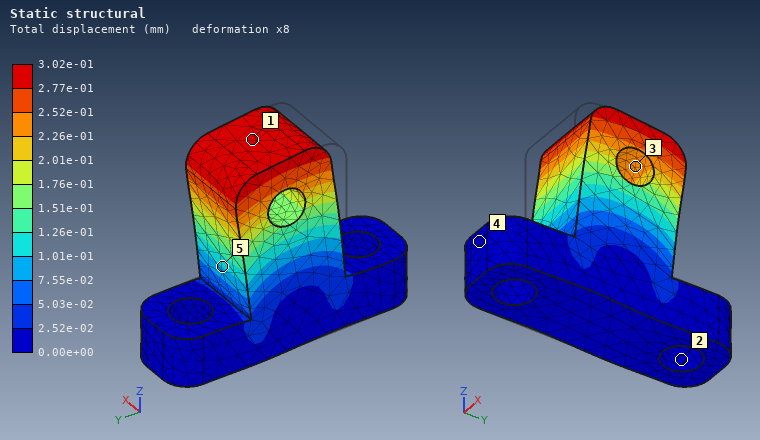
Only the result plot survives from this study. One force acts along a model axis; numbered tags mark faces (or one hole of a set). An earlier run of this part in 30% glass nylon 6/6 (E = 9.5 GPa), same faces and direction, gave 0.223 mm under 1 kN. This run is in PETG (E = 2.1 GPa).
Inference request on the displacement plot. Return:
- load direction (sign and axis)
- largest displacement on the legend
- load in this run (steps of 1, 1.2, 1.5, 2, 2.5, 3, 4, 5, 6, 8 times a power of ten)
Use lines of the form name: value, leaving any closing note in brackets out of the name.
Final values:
load direction: +Y
largest displacement on the legend: 3.02e-01 mm
load in this run: 300 N
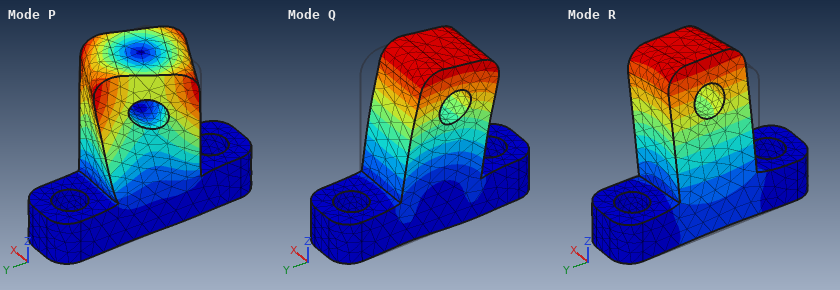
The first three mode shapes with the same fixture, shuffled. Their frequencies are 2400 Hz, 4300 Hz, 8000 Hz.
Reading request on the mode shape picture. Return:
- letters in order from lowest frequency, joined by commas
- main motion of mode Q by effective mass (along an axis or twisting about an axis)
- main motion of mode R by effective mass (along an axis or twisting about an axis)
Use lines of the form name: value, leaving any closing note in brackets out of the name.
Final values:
letters in order from lowest frequency, joined by commas: R, Q, P
main motion of mode Q by effective mass: along Y
main motion of mode R by effective mass: along X
